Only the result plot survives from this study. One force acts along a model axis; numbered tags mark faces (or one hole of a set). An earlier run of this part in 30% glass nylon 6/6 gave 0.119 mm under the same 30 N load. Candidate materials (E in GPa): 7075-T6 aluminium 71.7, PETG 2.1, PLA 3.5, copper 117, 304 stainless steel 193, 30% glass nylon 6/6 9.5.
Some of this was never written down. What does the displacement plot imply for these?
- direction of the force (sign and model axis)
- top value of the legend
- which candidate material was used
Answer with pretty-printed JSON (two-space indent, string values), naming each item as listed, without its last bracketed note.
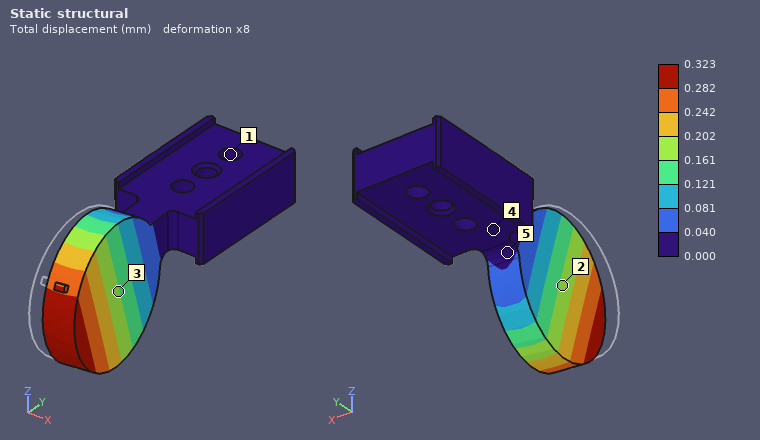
{
  "direction of the force": "+X",
  "top value of the legend": "0.323 mm",
  "which candidate material was used": "PLA"
}
